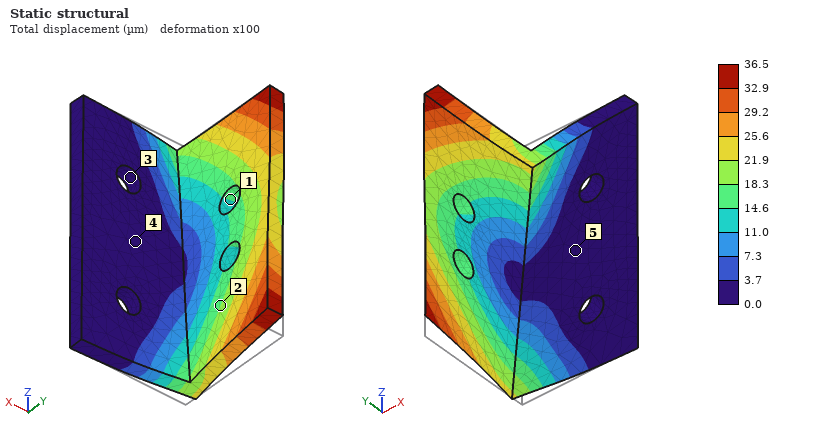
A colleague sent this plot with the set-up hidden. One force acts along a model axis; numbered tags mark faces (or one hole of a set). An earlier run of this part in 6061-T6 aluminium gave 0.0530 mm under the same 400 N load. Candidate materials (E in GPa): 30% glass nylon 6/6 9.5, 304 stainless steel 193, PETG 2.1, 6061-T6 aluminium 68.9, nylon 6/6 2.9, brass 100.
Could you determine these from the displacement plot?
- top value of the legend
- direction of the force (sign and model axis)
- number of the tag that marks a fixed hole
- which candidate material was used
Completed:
36.5 µm
+Z
3
brass
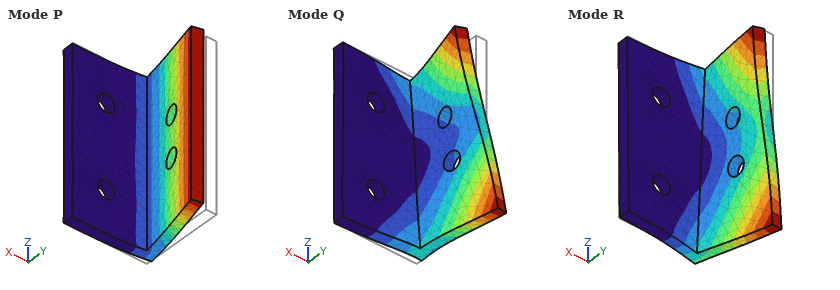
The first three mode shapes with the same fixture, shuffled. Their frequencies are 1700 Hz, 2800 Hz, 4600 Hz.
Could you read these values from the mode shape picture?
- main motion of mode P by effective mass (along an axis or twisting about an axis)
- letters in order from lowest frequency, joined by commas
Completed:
along X
P, R, Q
